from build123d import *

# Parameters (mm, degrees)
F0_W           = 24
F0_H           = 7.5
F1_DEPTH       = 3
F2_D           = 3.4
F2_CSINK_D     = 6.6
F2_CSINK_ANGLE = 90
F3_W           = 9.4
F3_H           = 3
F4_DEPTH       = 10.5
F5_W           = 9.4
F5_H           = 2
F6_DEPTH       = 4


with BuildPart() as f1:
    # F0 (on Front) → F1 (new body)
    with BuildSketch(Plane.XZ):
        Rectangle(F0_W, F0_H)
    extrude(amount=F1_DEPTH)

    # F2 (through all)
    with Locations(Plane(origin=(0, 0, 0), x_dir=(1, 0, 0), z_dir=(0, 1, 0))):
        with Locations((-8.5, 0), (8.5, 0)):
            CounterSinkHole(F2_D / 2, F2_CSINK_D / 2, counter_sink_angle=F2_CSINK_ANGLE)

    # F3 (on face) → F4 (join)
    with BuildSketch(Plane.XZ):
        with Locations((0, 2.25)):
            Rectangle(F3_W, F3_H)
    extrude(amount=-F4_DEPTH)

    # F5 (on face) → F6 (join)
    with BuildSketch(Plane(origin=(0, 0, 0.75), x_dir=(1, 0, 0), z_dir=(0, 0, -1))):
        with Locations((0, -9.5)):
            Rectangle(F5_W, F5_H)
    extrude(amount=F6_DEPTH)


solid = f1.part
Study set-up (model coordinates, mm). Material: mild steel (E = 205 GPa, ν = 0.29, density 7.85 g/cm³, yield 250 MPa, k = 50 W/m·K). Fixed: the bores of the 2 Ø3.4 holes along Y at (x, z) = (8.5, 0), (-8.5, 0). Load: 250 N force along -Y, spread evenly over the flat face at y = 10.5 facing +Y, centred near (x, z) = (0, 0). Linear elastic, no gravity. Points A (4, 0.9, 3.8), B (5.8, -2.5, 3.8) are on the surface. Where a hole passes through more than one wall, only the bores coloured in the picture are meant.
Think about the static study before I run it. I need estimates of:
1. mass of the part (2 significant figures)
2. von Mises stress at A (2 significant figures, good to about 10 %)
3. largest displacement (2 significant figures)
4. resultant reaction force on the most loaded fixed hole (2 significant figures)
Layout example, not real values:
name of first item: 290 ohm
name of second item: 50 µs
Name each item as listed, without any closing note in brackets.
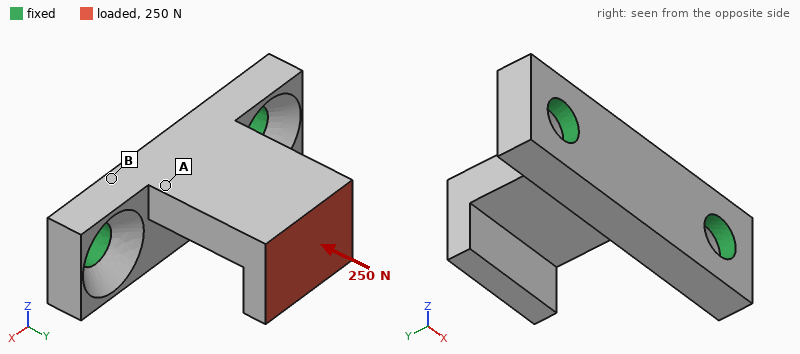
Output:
mass of the part: 6.4 g
von Mises stress at A: 23 MPa
largest displacement: 13 µm
resultant reaction force on the most loaded fixed hole: 150 N
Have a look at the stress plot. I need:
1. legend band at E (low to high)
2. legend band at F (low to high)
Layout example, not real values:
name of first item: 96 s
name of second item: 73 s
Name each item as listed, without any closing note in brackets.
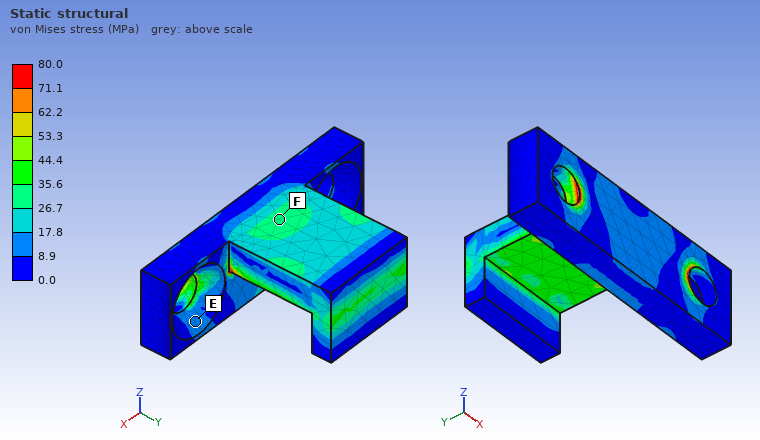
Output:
legend band at E: 8.9 to 17.8 MPa
legend band at F: 26.7 to 35.6 MPa
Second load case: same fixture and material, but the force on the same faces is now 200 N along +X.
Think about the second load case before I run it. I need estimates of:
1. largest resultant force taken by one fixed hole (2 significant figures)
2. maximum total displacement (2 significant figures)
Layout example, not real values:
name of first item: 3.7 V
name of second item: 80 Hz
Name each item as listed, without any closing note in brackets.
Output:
largest resultant force taken by one fixed hole: 210 N
maximum total displacement: 12 µm
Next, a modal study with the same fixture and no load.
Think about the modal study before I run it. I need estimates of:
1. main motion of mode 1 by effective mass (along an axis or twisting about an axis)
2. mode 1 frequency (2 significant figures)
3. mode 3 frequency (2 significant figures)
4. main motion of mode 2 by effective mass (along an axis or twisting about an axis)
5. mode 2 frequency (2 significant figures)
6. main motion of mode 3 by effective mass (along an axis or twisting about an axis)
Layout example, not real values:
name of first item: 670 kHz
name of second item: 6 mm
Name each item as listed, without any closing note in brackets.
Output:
main motion of mode 1 by effective mass: along Z
mode 1 frequency: 8600 Hz
mode 3 frequency: 29 kHz
main motion of mode 2 by effective mass: along X
mode 2 frequency: 20 kHz
main motion of mode 3 by effective mass: along Y
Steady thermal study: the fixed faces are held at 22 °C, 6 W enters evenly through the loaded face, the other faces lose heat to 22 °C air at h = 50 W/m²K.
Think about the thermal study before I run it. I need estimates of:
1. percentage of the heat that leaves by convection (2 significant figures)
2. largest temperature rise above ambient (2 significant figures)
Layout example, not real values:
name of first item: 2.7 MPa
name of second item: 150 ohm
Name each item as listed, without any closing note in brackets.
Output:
percentage of the heat that leaves by convection: 13 %
largest temperature rise above ambient: 64 K
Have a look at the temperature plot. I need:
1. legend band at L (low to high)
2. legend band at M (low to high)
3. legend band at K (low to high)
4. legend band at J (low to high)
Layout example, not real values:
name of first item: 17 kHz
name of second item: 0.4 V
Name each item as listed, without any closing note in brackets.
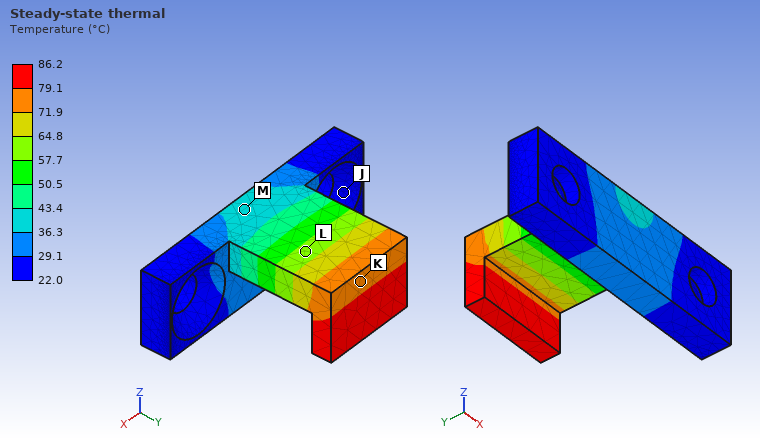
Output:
legend band at L: 57.7 to 64.8 °C
legend band at M: 36.3 to 43.4 °C
legend band at K: 71.9 to 79.1 °C
legend band at J: 22.0 to 29.1 °C
